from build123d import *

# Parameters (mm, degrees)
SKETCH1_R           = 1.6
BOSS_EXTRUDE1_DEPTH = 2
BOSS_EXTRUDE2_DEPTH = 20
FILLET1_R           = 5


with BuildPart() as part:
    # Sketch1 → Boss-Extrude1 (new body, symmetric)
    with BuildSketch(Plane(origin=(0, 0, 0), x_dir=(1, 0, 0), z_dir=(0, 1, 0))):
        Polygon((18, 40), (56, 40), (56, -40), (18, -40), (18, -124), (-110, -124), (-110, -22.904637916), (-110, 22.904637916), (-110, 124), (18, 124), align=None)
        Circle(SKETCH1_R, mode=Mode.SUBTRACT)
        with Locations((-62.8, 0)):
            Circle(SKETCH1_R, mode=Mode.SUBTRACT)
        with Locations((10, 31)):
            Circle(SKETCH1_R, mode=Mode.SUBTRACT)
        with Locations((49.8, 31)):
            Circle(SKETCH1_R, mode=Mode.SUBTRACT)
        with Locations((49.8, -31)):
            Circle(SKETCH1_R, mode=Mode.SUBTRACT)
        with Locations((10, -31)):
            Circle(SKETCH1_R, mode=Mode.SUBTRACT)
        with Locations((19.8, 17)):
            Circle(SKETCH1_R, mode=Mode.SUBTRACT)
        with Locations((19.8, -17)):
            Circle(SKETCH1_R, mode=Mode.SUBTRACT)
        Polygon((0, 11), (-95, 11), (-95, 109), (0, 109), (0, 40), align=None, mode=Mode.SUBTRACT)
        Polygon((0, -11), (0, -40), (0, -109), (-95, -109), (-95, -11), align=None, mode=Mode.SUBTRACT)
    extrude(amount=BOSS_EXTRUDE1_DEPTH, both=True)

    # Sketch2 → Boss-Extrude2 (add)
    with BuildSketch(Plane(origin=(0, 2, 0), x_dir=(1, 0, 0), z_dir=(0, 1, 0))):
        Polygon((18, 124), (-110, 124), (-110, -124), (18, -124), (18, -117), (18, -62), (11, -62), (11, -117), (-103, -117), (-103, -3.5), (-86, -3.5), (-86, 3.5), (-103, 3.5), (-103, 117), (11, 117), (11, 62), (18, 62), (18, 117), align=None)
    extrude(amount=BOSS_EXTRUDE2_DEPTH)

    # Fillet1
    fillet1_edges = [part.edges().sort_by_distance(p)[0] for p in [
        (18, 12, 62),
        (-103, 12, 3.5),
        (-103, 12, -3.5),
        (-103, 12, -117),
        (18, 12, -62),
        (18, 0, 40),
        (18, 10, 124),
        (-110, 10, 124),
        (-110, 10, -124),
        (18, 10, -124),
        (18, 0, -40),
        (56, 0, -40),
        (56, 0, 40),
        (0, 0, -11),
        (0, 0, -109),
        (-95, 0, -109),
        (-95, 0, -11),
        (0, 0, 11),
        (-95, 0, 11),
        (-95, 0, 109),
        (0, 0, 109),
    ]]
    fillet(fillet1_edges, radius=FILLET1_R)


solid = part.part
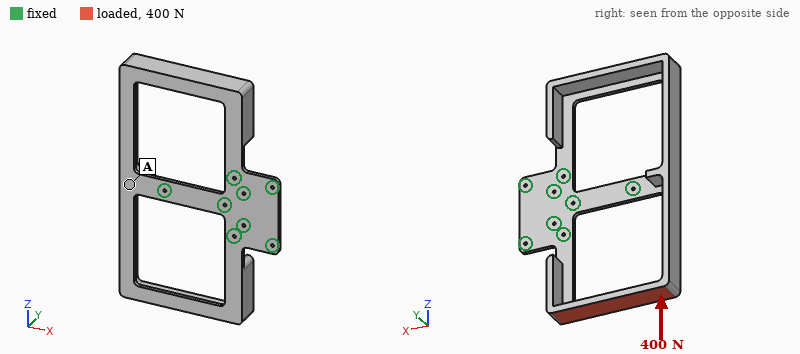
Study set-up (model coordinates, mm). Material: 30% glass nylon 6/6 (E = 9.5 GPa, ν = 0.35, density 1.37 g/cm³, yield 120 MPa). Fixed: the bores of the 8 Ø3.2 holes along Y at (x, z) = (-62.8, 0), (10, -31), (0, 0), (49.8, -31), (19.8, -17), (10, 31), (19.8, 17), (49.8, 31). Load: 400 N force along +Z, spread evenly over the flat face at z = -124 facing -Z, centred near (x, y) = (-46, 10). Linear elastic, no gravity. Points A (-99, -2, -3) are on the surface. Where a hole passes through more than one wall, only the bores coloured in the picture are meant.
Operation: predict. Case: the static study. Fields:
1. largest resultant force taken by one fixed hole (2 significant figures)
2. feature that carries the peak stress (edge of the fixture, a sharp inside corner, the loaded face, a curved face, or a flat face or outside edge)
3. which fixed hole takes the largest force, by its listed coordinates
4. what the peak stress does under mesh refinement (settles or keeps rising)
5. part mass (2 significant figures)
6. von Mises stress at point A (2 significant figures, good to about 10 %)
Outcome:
290 N
edge of the fixture
(-62.8, 0)
keeps rising
210 g
4.0 MPa
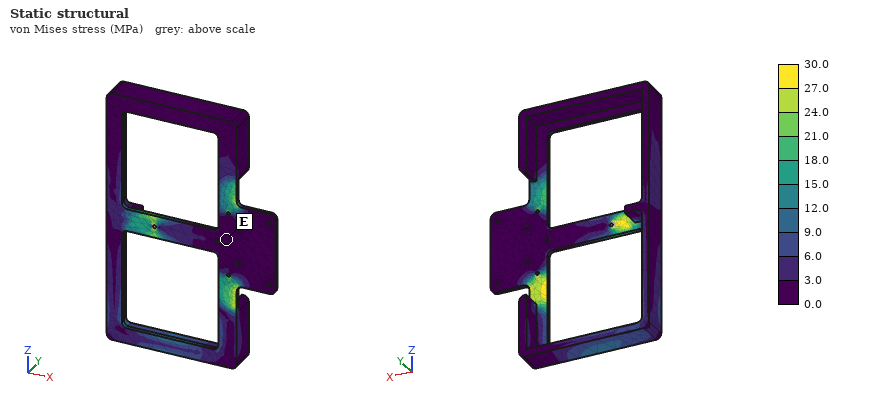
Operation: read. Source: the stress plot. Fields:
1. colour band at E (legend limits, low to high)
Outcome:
0.0 to 3.0 MPa
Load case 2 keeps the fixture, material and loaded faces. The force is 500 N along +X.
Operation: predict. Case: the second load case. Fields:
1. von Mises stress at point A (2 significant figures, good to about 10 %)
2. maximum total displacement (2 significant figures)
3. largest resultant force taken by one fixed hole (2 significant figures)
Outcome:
9.1 MPa
3.4 mm
410 N
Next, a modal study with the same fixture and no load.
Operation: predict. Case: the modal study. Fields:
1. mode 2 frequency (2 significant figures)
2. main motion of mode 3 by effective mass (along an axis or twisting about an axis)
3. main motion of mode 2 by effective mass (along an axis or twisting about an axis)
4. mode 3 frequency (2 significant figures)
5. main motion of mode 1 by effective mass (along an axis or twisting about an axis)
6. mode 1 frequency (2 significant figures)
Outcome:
160 Hz
along Y
along Y
180 Hz
twisting about X
60 Hz
